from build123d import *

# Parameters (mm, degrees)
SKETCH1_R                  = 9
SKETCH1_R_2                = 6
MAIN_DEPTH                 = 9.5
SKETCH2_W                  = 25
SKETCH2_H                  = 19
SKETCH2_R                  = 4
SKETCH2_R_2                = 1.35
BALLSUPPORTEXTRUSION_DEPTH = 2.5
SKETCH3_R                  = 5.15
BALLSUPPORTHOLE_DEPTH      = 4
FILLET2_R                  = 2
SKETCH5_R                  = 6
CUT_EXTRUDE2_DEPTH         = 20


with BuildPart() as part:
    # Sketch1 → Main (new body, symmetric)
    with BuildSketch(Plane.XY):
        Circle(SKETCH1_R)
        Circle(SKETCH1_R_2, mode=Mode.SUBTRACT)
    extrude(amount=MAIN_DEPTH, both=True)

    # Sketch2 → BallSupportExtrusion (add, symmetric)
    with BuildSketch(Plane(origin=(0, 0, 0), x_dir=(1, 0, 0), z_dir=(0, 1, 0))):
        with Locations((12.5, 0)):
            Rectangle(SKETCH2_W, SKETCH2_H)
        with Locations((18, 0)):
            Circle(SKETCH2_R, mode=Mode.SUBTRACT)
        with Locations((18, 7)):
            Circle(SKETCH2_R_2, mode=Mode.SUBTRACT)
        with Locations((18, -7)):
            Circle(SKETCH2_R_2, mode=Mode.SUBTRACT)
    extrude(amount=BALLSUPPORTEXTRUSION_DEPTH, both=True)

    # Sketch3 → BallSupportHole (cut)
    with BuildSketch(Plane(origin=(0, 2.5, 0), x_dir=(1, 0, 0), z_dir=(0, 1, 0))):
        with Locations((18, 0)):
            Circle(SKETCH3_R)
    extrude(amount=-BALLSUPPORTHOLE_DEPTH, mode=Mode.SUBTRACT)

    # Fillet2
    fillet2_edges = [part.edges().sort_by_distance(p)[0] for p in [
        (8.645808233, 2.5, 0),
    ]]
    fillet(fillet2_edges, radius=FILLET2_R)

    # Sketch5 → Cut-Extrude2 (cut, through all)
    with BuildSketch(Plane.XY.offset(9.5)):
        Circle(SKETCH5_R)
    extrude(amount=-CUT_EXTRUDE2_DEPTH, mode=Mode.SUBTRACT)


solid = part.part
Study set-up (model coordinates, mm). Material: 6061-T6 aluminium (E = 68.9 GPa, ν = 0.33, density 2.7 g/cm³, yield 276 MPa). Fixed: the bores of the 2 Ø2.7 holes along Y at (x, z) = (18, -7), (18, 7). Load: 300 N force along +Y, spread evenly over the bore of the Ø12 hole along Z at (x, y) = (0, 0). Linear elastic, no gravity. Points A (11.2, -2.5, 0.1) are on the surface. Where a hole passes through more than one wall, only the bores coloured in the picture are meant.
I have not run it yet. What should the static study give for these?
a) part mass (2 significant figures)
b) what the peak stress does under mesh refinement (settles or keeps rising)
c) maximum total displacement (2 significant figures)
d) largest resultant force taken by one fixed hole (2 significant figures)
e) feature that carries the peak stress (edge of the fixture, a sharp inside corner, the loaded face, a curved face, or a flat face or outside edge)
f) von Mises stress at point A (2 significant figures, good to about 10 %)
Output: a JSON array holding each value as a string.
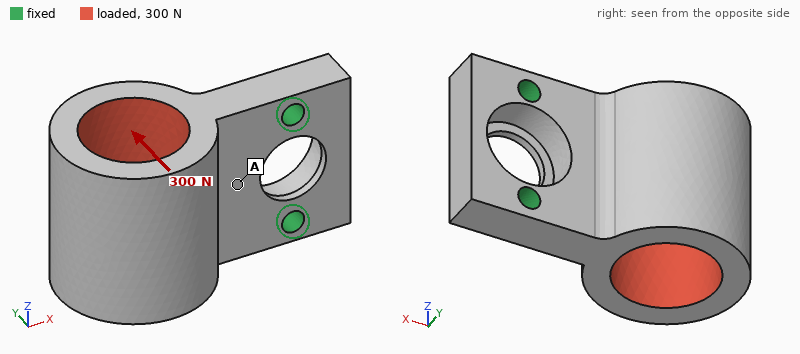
["10 g", "keeps rising", "0.11 mm", "150 N", "edge of the fixture", "19 MPa"]
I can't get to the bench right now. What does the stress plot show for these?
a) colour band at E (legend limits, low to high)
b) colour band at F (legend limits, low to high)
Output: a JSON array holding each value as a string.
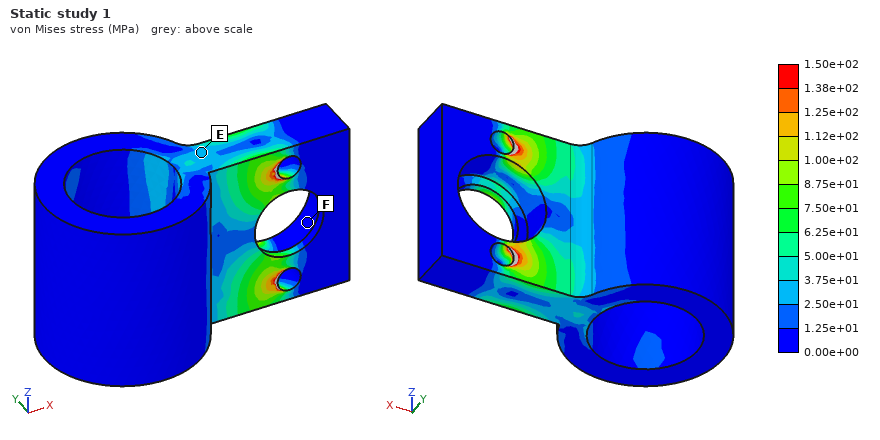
["2.50e+01 to 3.75e+01 MPa", "0.00e+00 to 1.25e+01 MPa"]
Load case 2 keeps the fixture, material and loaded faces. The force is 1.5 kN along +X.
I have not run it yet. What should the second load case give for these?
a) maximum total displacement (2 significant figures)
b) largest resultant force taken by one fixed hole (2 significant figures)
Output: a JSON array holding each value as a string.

["17 µm", "770 N"]
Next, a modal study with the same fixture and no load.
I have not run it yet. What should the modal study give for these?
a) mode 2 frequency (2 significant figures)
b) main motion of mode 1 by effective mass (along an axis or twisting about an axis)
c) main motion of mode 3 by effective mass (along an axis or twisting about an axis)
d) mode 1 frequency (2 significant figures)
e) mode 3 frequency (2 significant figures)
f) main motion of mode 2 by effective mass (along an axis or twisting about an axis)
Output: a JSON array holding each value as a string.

["11 kHz", "along Y", "twisting about X", "3500 Hz", "13 kHz", "along Z"]
